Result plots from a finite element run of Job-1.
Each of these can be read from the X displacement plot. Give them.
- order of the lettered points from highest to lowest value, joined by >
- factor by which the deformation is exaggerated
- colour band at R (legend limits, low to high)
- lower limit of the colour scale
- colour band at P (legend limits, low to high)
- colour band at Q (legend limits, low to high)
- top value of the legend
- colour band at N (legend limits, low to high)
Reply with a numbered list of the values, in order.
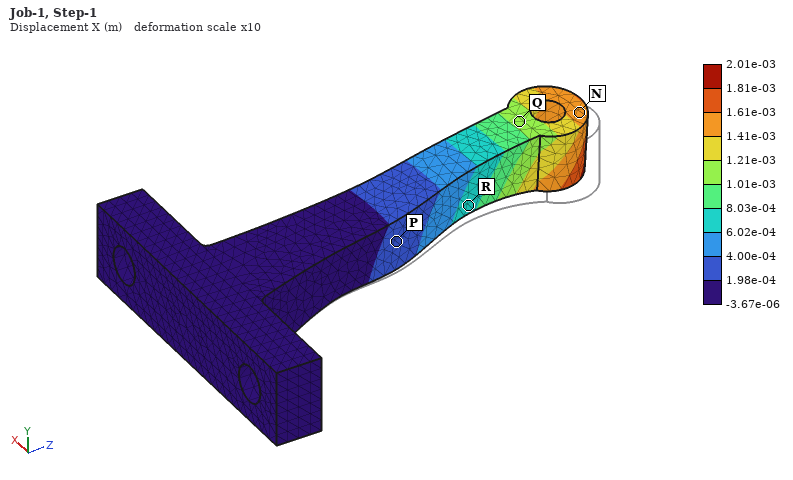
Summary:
1. N > Q > R > P
2. 10
3. 6.02e-04 to 8.03e-04 m
4. -3.67e-06 m
5. 1.98e-04 to 4.00e-04 m
6. 1.01e-03 to 1.21e-03 m
7. 2.01e-03 m
8. 1.41e-03 to 1.61e-03 m
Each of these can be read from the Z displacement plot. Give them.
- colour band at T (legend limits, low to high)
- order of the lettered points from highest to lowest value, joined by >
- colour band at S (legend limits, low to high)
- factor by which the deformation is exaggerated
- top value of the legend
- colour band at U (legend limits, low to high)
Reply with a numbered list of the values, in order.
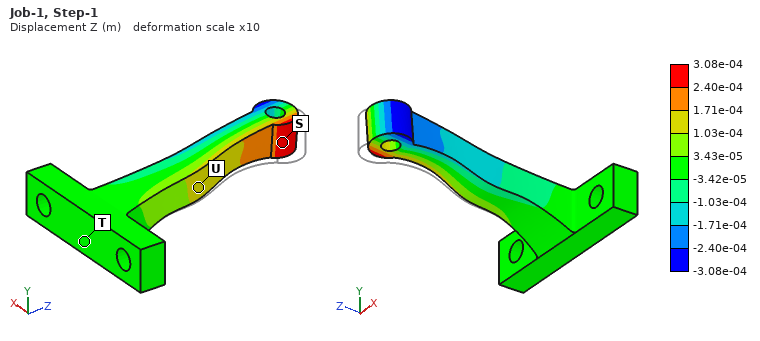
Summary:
1. -3.42e-05 to 3.43e-05 m
2. S > U > T
3. 2.40e-04 to 3.08e-04 m
4. 10
5. 3.08e-04 m
6. 1.03e-04 to 1.71e-04 m
